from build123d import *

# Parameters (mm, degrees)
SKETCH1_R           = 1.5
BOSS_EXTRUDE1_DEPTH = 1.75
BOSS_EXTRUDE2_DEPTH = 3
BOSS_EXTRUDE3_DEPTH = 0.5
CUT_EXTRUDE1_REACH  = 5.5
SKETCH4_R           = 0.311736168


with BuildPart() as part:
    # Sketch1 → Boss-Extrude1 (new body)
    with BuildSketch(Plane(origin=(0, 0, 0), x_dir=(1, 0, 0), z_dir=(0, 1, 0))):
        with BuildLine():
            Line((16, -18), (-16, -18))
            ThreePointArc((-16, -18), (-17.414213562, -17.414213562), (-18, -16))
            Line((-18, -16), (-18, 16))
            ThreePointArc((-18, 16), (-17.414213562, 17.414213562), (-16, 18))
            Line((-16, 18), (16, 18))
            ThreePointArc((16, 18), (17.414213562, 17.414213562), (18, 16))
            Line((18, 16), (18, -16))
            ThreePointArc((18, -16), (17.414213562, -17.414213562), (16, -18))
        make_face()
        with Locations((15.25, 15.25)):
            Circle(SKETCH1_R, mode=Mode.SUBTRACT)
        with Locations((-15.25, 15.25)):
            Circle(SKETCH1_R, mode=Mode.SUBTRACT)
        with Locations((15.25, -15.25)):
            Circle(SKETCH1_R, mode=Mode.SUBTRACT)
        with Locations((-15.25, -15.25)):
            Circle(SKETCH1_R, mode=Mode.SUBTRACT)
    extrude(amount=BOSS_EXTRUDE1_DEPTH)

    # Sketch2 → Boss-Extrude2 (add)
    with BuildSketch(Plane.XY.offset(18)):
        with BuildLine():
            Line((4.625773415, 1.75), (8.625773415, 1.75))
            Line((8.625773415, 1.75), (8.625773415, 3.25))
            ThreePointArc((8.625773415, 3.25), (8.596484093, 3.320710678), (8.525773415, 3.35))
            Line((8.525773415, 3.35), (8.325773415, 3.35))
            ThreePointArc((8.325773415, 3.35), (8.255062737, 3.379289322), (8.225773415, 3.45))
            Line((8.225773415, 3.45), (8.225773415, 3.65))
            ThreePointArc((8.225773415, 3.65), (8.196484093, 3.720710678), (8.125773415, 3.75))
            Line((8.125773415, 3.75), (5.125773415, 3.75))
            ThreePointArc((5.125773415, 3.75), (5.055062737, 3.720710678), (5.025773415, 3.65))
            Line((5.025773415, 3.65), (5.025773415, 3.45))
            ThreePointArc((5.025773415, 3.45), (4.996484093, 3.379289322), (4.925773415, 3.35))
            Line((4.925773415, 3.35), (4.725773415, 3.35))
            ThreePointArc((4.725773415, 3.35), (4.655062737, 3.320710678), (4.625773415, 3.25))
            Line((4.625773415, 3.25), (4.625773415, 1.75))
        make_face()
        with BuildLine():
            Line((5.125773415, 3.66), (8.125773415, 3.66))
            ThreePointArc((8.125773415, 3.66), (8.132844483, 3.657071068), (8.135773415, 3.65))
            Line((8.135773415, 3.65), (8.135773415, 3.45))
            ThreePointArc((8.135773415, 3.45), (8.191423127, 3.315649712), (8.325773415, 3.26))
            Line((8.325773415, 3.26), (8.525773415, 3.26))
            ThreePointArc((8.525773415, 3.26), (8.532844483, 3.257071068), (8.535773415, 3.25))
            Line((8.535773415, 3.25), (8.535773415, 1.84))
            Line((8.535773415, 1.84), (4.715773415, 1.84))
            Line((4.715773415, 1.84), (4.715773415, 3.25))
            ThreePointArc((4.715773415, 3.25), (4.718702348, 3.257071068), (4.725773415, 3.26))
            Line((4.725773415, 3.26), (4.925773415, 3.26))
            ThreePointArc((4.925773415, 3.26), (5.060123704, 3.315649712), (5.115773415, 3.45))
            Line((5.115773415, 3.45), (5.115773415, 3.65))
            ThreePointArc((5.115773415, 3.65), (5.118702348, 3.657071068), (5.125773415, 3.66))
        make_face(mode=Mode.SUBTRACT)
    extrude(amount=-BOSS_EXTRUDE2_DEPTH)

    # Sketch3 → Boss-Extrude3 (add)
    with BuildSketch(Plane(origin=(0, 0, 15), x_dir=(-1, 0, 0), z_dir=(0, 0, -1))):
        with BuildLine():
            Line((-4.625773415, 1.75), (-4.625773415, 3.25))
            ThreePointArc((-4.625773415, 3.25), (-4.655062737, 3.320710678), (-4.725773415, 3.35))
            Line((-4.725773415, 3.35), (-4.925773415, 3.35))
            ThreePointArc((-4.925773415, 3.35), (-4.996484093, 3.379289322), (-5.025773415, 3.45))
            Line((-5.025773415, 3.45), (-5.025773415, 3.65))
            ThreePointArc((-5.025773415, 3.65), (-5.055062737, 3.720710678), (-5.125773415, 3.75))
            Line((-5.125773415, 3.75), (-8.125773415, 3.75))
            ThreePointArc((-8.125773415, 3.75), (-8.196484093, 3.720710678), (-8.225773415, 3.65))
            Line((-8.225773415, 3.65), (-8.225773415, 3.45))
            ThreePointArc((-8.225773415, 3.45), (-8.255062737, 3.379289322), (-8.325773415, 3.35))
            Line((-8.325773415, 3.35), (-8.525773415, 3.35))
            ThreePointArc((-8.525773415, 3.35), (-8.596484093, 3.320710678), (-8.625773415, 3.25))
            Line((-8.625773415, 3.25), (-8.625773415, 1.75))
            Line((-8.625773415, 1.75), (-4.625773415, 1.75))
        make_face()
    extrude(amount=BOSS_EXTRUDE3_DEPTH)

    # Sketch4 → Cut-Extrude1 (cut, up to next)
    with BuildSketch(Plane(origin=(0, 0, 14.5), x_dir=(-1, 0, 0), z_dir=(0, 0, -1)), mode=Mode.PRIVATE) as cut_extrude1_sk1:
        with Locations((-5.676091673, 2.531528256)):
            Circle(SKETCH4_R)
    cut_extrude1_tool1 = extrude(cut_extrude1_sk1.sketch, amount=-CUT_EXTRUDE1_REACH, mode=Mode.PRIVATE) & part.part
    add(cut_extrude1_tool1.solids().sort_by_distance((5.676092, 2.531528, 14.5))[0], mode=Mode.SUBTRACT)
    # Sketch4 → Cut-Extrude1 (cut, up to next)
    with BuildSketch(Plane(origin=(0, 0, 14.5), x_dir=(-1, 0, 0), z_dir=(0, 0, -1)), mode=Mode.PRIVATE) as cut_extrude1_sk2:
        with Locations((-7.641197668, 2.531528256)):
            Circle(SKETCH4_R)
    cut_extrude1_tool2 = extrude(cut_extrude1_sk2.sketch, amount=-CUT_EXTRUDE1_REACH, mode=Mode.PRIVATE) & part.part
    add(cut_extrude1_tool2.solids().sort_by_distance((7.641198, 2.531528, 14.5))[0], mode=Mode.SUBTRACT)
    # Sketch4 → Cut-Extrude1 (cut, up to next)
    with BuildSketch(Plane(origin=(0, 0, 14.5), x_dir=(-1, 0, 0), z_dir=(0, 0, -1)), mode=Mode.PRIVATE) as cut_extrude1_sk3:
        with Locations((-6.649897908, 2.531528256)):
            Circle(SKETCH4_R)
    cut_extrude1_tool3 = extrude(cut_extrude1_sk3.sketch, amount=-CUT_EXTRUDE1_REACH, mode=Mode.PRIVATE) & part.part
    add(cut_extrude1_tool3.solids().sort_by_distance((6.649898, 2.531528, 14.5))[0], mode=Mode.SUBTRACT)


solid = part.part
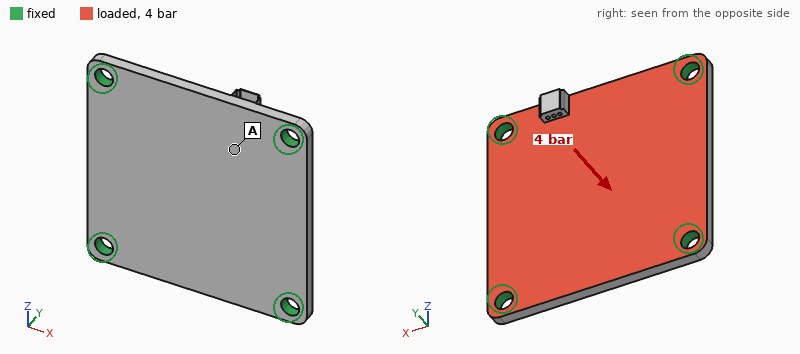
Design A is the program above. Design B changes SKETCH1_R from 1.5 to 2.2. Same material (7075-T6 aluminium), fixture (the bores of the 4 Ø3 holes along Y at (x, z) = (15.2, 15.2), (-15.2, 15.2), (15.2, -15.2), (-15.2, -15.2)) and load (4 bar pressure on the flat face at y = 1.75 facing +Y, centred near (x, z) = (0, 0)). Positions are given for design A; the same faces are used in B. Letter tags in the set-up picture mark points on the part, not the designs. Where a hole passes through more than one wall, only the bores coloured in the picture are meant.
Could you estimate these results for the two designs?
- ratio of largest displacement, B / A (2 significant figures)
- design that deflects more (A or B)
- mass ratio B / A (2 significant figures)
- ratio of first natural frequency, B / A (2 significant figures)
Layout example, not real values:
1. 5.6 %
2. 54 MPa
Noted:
1. 0.82
2. A
3. 0.97
4. 1.1
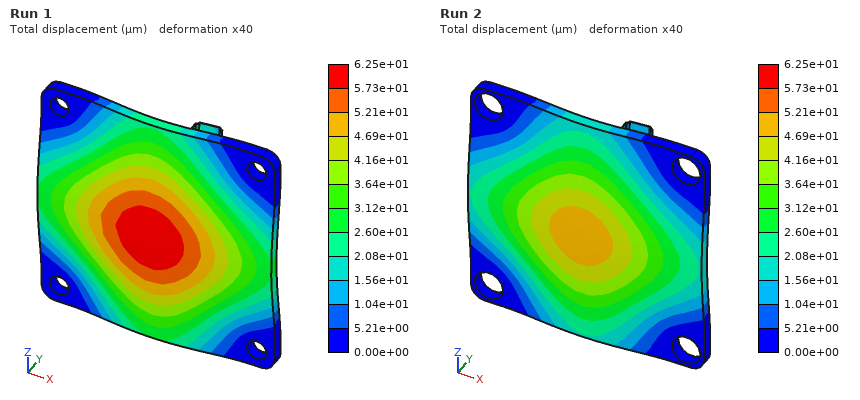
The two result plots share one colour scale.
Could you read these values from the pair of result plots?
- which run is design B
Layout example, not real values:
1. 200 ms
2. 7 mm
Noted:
1. Run 2
